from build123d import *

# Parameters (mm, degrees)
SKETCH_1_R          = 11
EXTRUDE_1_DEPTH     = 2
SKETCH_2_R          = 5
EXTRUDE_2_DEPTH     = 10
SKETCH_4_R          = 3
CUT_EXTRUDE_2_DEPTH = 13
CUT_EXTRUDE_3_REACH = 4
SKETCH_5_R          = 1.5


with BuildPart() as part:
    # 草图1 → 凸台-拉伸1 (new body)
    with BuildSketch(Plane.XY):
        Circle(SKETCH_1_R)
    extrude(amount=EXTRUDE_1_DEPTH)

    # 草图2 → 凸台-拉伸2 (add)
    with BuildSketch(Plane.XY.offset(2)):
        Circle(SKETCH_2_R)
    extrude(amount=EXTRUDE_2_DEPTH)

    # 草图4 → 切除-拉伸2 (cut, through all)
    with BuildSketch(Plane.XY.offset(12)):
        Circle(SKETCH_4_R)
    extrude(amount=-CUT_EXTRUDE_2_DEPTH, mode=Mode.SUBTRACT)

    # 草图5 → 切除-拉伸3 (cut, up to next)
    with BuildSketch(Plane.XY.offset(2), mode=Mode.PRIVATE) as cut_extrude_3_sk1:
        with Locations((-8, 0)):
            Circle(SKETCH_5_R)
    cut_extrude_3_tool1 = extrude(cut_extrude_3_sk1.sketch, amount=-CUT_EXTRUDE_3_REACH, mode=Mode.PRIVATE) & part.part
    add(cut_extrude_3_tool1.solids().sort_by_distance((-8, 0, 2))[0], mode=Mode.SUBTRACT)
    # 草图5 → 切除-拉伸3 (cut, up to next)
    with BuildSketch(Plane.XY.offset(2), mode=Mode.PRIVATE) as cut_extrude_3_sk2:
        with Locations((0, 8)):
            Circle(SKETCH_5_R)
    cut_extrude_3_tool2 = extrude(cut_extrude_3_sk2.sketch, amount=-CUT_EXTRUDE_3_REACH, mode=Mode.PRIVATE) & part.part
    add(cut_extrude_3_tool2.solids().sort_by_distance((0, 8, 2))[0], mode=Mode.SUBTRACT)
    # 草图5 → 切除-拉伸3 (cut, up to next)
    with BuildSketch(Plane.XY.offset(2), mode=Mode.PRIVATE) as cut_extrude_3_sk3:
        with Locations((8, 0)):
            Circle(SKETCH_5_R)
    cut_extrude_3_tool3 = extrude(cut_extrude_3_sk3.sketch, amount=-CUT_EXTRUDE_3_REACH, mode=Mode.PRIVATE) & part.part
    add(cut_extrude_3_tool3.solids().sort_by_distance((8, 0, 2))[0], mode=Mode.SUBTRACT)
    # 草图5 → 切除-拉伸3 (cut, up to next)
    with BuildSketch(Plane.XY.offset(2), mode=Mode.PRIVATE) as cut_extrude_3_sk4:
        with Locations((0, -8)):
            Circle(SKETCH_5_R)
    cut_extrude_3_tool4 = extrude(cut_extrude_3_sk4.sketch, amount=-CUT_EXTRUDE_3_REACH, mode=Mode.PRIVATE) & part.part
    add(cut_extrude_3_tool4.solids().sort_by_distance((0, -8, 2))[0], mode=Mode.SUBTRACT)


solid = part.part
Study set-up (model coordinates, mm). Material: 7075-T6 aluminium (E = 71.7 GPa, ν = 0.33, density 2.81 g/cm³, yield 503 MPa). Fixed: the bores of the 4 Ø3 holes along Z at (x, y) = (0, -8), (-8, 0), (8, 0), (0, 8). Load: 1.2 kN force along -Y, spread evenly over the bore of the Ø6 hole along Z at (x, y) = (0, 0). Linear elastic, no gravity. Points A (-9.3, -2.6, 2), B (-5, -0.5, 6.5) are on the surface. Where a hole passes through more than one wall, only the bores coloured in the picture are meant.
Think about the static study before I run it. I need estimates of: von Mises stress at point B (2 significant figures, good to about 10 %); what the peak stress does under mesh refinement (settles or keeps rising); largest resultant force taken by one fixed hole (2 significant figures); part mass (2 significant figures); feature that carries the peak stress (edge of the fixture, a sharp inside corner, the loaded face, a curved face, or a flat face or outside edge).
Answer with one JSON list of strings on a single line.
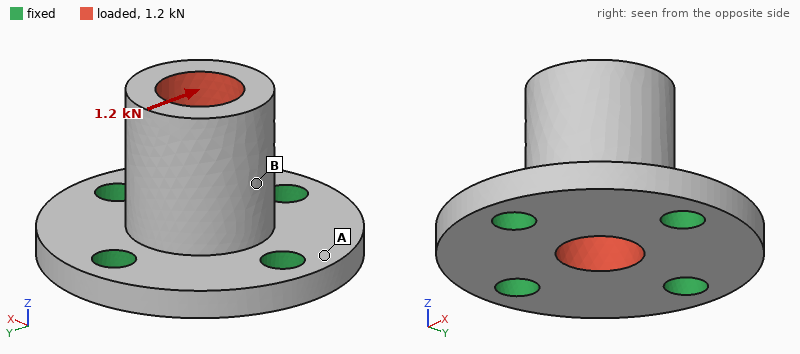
["28 MPa", "keeps rising", "600 N", "3.2 g", "edge of the fixture"]
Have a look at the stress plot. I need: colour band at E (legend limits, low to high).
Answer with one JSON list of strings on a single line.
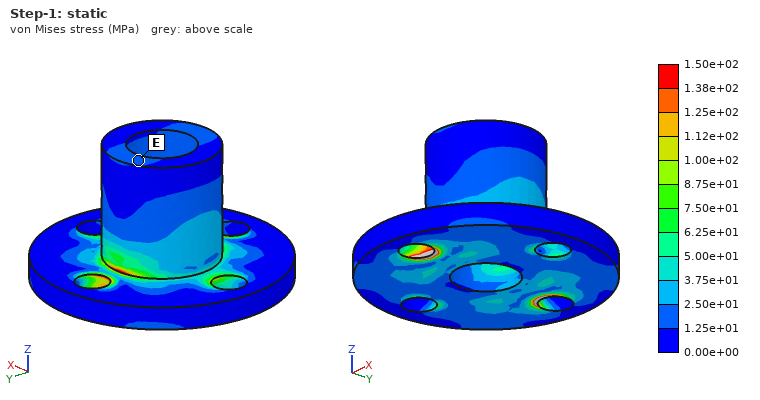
["1.25e+01 to 2.50e+01 MPa"]
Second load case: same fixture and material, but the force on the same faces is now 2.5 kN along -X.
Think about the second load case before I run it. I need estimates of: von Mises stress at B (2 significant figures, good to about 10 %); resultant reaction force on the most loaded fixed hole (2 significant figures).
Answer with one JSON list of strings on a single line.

["28 MPa", "1.3 kN"]
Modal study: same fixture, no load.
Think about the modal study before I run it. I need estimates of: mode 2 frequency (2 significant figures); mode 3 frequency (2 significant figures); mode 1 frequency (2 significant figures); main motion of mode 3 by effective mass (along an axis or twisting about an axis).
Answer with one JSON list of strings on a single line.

["30 kHz", "53 kHz", "30 kHz", "along Z"]
